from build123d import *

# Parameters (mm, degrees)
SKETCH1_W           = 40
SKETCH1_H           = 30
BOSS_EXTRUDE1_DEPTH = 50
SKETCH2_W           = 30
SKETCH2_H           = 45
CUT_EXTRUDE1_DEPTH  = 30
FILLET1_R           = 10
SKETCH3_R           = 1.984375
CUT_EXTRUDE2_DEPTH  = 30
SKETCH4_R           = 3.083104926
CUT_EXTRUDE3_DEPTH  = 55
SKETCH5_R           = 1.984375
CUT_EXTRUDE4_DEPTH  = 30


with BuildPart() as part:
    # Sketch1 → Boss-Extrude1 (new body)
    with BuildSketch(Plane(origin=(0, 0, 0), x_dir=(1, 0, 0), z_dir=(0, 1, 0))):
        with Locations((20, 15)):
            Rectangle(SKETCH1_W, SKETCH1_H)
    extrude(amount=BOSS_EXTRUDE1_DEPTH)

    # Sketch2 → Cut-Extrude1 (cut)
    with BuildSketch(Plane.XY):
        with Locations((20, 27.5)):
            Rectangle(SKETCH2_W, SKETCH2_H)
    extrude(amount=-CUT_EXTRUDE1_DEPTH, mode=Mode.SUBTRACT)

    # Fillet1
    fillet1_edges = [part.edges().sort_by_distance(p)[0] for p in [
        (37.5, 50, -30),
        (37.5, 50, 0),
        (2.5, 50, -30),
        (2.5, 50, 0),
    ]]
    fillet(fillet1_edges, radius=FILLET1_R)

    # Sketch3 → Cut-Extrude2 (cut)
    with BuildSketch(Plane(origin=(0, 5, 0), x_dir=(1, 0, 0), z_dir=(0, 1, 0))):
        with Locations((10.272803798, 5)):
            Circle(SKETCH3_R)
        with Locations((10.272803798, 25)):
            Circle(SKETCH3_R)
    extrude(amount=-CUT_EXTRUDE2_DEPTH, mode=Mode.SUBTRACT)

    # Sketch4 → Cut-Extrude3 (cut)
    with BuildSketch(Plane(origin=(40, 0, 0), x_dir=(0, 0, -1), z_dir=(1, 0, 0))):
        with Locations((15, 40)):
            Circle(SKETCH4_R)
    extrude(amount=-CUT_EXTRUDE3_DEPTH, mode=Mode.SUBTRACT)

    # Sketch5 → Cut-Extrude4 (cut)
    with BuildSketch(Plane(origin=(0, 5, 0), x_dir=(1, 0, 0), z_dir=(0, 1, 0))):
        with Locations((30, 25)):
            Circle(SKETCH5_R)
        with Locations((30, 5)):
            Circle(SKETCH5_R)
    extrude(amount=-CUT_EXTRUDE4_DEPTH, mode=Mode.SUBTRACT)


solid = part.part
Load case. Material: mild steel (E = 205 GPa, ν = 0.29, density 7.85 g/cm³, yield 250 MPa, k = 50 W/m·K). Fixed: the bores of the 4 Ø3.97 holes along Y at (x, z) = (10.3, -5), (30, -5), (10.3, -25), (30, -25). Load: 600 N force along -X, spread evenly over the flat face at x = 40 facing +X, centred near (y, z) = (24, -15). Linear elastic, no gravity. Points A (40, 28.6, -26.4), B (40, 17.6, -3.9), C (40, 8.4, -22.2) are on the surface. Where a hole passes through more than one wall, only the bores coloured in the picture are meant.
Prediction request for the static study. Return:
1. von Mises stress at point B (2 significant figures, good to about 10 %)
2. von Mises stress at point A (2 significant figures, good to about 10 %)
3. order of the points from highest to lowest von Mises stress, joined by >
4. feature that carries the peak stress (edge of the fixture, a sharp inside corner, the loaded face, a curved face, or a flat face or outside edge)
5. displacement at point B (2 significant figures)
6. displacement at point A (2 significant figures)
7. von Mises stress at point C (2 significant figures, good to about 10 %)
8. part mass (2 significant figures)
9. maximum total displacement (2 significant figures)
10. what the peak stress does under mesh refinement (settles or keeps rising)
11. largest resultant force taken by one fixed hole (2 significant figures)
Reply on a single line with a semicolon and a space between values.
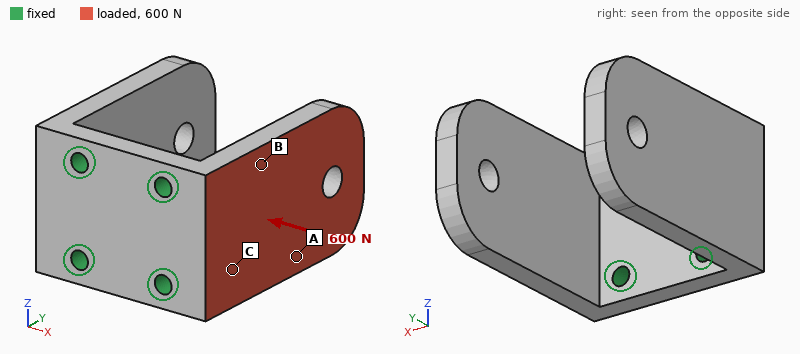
47 MPa; 20 MPa; C > B > A; edge of the fixture; 0.037 mm; 0.075 mm; 73 MPa; 150 g; 0.16 mm; keeps rising; 270 N
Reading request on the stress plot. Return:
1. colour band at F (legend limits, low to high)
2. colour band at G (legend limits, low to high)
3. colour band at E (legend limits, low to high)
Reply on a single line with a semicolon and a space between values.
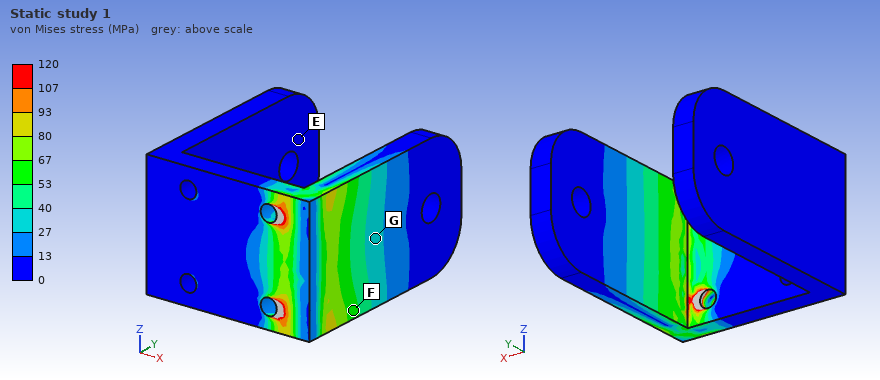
53 to 67 MPa; 27 to 40 MPa; 0 to 13 MPa
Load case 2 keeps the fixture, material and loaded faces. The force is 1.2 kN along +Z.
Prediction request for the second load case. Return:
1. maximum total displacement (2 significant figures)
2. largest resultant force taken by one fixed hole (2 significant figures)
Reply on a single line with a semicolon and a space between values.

26 µm; 1.4 kN
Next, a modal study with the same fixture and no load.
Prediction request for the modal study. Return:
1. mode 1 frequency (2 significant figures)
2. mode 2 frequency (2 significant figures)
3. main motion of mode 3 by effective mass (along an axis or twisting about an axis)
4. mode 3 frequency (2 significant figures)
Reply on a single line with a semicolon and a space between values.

1600 Hz; 1600 Hz; along Z; 5000 Hz
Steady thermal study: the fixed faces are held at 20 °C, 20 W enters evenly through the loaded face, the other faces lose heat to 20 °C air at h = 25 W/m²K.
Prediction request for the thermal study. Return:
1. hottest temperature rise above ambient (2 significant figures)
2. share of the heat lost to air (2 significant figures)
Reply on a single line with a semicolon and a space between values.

63 K; 13 %
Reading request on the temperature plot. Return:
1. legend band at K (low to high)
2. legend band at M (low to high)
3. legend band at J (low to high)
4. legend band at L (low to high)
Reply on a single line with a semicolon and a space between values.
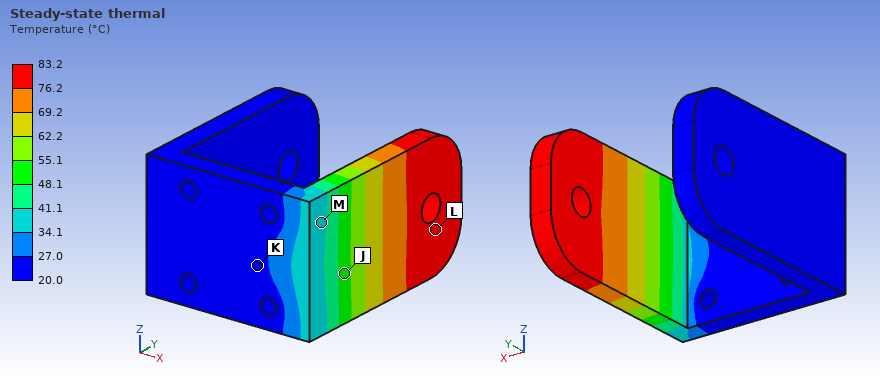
20.0 to 27.0 °C; 34.1 to 41.1 °C; 48.1 to 55.1 °C; 76.2 to 83.2 °C
